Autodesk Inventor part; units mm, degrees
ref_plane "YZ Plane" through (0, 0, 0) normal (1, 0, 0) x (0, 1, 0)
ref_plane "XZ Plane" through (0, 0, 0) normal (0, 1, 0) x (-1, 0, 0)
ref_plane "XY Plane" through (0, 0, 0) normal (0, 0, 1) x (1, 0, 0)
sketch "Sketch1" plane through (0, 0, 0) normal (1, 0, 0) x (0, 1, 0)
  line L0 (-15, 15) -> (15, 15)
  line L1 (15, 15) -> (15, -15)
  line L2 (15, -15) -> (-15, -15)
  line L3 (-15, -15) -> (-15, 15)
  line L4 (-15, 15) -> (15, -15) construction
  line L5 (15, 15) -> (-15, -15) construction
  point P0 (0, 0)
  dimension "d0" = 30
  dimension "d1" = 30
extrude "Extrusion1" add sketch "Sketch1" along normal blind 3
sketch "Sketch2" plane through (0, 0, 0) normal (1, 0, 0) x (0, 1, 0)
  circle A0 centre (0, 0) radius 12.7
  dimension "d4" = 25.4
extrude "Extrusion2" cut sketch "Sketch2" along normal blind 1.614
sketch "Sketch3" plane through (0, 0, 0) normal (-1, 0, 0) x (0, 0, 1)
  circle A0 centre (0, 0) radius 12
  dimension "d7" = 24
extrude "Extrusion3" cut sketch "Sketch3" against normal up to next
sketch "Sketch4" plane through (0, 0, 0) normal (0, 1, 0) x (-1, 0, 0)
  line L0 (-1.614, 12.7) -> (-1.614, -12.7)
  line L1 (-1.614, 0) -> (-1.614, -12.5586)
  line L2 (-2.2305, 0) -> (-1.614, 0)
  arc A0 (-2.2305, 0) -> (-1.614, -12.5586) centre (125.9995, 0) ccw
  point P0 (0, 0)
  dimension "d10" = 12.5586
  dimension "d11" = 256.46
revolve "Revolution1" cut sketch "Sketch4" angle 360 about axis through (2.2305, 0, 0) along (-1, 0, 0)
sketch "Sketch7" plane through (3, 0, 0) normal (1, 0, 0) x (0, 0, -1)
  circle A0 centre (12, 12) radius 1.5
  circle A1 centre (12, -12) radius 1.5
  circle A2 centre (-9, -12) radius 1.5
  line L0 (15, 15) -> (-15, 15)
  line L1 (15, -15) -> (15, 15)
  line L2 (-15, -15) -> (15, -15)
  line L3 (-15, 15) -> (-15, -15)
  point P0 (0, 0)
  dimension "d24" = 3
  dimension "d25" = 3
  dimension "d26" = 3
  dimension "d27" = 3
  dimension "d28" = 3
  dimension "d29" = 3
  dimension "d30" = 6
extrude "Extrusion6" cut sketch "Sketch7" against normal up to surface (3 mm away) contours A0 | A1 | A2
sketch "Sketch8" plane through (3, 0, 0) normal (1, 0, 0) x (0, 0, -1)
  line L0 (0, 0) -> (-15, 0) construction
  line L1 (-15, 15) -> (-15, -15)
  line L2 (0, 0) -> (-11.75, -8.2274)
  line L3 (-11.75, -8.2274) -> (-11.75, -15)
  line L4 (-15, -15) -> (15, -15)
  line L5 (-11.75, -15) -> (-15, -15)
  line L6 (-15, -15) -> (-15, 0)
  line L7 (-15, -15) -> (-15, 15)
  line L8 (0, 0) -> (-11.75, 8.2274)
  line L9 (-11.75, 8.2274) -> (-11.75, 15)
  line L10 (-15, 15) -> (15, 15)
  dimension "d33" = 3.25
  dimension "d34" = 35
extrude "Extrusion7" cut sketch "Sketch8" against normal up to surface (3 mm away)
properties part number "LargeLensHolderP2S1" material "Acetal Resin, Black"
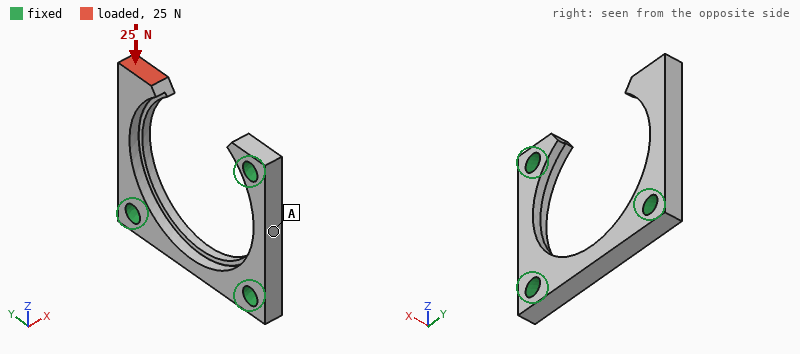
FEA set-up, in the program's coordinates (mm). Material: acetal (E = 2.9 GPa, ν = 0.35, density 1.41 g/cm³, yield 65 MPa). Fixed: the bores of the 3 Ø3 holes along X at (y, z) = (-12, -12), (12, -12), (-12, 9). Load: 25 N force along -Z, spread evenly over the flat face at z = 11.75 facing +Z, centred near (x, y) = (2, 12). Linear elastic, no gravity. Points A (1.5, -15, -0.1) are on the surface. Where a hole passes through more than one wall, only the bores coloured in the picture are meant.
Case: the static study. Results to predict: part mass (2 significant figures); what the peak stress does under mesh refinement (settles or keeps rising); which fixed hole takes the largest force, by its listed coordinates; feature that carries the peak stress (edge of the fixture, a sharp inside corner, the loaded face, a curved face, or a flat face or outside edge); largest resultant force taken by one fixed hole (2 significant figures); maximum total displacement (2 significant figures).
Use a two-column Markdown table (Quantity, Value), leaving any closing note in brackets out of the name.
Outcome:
| Quantity | Value |
|---|---|
| part mass | 1.3 g |
| what the peak stress does under mesh refinement | keeps rising |
| which fixed hole takes the largest force, by its listed coordinates | (12, -12) |
| feature that carries the peak stress | a sharp inside corner |
| largest resultant force taken by one fixed hole | 25 N |
| maximum total displacement | 0.42 mm |
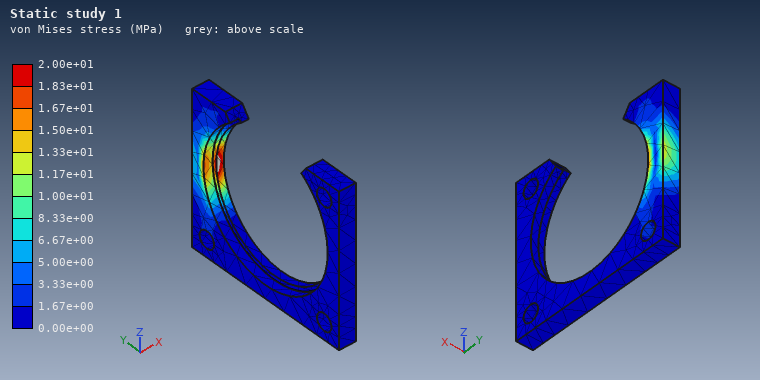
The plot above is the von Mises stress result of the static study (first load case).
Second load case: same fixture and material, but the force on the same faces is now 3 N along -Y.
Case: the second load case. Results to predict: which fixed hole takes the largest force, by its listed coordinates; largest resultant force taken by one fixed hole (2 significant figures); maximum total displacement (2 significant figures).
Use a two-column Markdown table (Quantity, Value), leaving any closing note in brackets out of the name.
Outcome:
| Quantity | Value |
|---|---|
| which fixed hole takes the largest force, by its listed coordinates | (12, -12) |
| largest resultant force taken by one fixed hole | 3.6 N |
| maximum total displacement | 0.37 mm |
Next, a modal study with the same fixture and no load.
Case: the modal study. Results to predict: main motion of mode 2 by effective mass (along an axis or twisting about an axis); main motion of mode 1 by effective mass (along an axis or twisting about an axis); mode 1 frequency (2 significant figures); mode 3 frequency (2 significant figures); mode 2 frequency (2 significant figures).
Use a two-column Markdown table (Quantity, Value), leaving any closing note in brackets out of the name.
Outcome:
| Quantity | Value |
|---|---|
| main motion of mode 2 by effective mass | along Y |
| main motion of mode 1 by effective mass | along X |
| mode 1 frequency | 1100 Hz |
| mode 3 frequency | 4800 Hz |
| mode 2 frequency | 1400 Hz |
